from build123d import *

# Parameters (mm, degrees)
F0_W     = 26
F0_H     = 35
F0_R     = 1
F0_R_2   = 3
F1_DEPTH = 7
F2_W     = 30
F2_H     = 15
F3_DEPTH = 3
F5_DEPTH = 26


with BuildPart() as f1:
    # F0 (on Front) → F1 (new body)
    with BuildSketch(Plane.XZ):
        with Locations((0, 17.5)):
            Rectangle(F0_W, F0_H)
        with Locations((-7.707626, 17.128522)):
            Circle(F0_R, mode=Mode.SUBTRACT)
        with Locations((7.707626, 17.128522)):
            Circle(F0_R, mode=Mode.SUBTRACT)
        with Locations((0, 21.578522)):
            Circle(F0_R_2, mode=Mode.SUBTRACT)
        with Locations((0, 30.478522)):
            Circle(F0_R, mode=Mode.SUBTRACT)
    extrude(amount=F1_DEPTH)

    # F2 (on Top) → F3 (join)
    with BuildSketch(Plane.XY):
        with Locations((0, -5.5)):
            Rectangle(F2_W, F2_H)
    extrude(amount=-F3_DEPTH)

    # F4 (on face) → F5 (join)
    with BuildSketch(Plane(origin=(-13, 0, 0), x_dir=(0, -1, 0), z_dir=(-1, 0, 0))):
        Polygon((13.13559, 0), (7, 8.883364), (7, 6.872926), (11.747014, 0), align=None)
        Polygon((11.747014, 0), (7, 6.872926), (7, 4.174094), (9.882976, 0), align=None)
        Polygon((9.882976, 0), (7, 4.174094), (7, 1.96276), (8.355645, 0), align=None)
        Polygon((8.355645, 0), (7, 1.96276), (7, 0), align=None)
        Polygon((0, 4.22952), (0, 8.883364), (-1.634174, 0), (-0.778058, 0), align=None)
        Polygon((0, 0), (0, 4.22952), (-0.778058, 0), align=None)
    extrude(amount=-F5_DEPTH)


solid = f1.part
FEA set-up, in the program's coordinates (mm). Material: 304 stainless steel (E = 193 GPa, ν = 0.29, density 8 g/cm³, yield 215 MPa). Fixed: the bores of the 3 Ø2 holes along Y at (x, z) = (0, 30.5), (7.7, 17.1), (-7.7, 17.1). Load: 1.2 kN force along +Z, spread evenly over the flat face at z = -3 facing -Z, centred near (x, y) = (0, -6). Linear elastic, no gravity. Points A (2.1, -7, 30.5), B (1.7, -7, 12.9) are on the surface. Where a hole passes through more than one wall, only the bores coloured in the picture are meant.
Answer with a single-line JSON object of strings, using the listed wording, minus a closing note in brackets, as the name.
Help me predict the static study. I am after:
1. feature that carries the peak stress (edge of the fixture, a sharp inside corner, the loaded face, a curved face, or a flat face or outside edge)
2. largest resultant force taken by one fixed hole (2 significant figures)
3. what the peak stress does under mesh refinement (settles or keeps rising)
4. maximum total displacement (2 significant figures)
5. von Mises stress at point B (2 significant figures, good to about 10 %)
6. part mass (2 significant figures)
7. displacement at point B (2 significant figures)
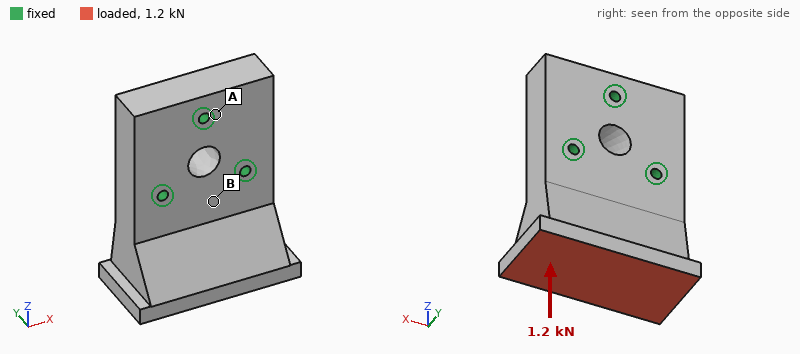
{"feature that carries the peak stress": "edge of the fixture", "largest resultant force taken by one fixed hole": "560 N", "what the peak stress does under mesh refinement": "keeps rising", "maximum total displacement": "4.5 µm", "von Mises stress at point B": "12 MPa", "part mass": "67 g", "displacement at point B": "0.76 µm"}
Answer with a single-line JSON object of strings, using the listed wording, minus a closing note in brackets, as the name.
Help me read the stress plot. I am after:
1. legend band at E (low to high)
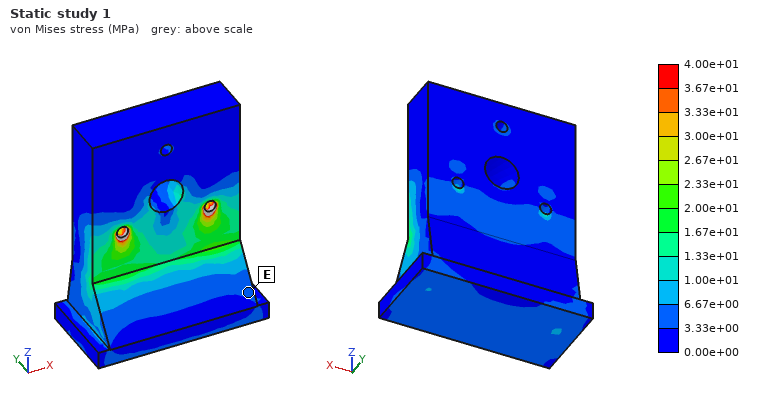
{"legend band at E": "3.33e+00 to 6.67e+00 MPa"}
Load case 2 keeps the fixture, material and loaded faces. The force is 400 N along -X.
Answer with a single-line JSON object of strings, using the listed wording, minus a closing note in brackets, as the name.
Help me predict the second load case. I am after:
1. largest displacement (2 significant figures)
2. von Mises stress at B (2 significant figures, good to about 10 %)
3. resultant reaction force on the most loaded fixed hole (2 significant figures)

{"largest displacement": "1.9 µm", "von Mises stress at B": "6.8 MPa", "resultant reaction force on the most loaded fixed hole": "490 N"}
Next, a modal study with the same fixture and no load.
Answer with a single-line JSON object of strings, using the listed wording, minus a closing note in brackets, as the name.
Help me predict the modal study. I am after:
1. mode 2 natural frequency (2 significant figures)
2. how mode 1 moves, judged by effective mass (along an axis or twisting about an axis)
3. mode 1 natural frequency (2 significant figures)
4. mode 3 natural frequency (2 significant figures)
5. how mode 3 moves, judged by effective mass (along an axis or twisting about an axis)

{"mode 2 natural frequency": "16 kHz", "how mode 1 moves, judged by effective mass": "along Y", "mode 1 natural frequency": "7700 Hz", "mode 3 natural frequency": "19 kHz", "how mode 3 moves, judged by effective mass": "along X"}
